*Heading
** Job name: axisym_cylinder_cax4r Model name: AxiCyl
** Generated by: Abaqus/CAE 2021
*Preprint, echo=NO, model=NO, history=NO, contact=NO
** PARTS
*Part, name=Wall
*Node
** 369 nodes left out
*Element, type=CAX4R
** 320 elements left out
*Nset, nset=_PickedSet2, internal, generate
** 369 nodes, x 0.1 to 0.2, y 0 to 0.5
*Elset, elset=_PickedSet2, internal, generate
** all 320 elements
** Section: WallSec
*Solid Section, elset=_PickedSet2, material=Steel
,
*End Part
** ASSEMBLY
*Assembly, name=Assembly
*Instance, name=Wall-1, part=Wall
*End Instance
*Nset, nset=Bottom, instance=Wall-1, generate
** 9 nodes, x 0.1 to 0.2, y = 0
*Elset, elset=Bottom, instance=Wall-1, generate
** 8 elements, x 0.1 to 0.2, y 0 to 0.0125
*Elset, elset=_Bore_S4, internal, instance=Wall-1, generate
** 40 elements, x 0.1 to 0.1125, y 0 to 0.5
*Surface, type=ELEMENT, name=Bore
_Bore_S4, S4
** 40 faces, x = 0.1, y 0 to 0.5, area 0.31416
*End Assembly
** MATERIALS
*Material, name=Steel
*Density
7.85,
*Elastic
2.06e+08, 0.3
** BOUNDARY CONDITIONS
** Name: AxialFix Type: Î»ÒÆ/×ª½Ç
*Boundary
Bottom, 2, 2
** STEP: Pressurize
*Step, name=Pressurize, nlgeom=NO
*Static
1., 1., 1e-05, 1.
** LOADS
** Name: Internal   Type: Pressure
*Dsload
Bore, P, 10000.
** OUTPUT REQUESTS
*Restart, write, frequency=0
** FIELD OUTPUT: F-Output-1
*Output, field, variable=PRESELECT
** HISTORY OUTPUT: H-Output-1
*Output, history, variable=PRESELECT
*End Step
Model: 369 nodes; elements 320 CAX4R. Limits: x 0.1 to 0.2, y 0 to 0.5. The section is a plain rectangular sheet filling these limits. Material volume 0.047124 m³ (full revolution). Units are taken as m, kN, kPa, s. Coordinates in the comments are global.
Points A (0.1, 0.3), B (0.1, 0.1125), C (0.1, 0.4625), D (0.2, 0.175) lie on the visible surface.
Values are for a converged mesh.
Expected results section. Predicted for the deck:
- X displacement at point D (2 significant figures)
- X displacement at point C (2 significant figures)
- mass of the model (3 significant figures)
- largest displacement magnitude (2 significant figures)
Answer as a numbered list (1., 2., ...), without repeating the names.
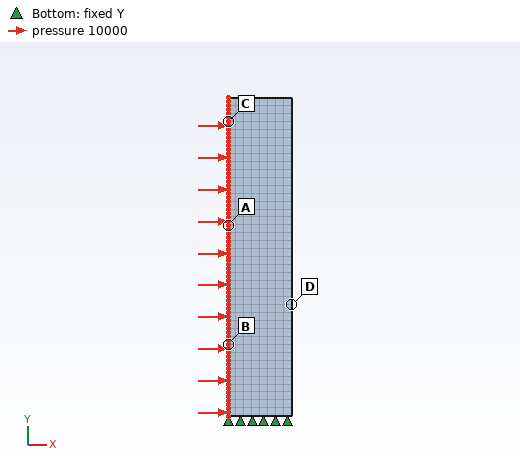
1. 6.5e-06 m
2. 9.5e-06 m
3. 370 kg
4. 1.1e-05 m
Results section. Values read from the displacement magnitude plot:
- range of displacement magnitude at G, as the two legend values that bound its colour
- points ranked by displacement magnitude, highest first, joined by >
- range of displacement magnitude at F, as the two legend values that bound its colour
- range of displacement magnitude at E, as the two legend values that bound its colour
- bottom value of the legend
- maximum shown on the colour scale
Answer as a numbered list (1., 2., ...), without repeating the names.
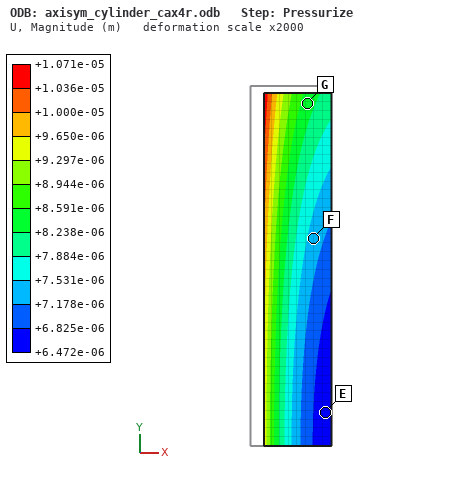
1. +8.238e-06 to +8.591e-06 m
2. G > F > E
3. +7.178e-06 to +7.531e-06 m
4. +6.472e-06 to +6.825e-06 m
5. +6.472e-06 m
6. +1.071e-05 m
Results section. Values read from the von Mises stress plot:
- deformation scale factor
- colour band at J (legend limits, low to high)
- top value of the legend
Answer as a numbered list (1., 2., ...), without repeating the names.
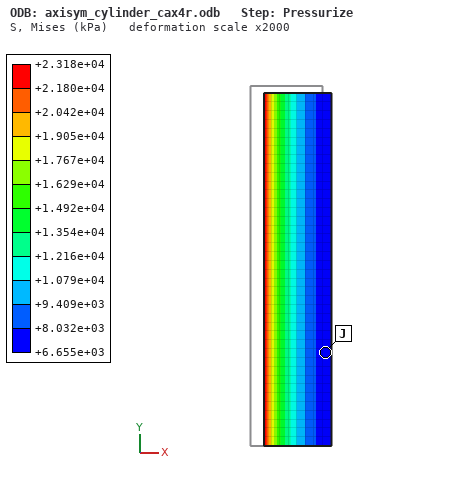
1. 2000
2. +6.655e+03 to +8.032e+03 kPa
3. +2.318e+04 kPa
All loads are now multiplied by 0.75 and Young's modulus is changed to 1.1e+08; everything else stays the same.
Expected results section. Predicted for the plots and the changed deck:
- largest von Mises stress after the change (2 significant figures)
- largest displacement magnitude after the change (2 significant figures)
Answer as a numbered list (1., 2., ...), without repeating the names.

1. 17000 kPa
2. 1.5e-05 m
